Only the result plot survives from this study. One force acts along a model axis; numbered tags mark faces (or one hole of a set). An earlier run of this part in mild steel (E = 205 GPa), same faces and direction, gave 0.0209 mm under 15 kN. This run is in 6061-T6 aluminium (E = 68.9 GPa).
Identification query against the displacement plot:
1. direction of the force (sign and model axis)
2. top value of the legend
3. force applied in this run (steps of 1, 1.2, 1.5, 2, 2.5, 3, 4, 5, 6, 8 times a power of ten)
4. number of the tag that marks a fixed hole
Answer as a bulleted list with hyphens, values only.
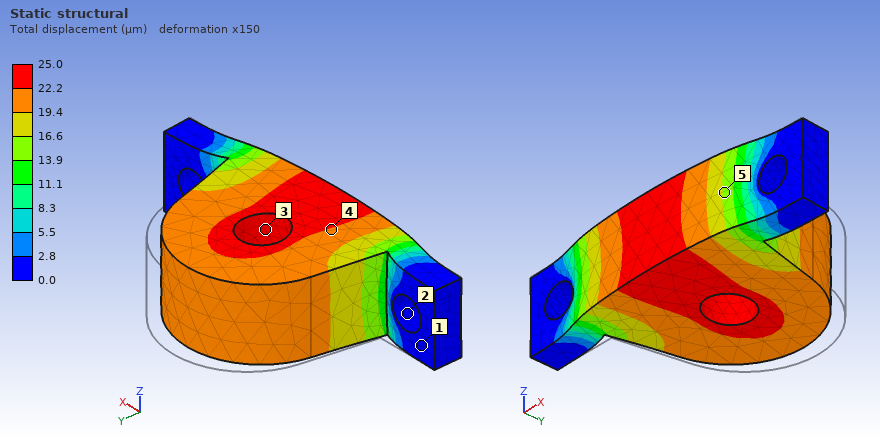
- -Y
- 25.0 µm
- 6 kN
- 2
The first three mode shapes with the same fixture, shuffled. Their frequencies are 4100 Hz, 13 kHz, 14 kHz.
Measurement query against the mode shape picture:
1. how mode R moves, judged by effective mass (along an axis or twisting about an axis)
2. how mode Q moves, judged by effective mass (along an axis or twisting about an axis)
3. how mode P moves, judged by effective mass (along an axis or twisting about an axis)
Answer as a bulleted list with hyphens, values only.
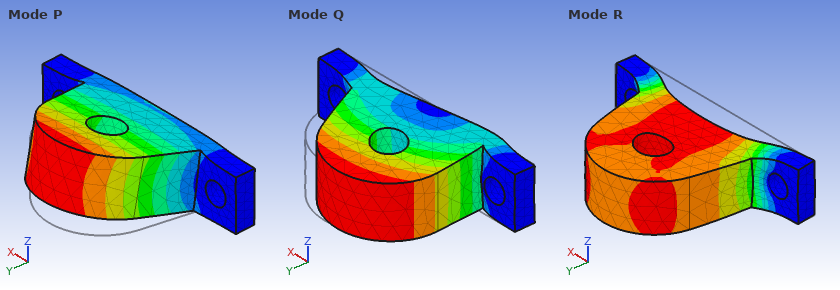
- along Y
- along X
- along Z
